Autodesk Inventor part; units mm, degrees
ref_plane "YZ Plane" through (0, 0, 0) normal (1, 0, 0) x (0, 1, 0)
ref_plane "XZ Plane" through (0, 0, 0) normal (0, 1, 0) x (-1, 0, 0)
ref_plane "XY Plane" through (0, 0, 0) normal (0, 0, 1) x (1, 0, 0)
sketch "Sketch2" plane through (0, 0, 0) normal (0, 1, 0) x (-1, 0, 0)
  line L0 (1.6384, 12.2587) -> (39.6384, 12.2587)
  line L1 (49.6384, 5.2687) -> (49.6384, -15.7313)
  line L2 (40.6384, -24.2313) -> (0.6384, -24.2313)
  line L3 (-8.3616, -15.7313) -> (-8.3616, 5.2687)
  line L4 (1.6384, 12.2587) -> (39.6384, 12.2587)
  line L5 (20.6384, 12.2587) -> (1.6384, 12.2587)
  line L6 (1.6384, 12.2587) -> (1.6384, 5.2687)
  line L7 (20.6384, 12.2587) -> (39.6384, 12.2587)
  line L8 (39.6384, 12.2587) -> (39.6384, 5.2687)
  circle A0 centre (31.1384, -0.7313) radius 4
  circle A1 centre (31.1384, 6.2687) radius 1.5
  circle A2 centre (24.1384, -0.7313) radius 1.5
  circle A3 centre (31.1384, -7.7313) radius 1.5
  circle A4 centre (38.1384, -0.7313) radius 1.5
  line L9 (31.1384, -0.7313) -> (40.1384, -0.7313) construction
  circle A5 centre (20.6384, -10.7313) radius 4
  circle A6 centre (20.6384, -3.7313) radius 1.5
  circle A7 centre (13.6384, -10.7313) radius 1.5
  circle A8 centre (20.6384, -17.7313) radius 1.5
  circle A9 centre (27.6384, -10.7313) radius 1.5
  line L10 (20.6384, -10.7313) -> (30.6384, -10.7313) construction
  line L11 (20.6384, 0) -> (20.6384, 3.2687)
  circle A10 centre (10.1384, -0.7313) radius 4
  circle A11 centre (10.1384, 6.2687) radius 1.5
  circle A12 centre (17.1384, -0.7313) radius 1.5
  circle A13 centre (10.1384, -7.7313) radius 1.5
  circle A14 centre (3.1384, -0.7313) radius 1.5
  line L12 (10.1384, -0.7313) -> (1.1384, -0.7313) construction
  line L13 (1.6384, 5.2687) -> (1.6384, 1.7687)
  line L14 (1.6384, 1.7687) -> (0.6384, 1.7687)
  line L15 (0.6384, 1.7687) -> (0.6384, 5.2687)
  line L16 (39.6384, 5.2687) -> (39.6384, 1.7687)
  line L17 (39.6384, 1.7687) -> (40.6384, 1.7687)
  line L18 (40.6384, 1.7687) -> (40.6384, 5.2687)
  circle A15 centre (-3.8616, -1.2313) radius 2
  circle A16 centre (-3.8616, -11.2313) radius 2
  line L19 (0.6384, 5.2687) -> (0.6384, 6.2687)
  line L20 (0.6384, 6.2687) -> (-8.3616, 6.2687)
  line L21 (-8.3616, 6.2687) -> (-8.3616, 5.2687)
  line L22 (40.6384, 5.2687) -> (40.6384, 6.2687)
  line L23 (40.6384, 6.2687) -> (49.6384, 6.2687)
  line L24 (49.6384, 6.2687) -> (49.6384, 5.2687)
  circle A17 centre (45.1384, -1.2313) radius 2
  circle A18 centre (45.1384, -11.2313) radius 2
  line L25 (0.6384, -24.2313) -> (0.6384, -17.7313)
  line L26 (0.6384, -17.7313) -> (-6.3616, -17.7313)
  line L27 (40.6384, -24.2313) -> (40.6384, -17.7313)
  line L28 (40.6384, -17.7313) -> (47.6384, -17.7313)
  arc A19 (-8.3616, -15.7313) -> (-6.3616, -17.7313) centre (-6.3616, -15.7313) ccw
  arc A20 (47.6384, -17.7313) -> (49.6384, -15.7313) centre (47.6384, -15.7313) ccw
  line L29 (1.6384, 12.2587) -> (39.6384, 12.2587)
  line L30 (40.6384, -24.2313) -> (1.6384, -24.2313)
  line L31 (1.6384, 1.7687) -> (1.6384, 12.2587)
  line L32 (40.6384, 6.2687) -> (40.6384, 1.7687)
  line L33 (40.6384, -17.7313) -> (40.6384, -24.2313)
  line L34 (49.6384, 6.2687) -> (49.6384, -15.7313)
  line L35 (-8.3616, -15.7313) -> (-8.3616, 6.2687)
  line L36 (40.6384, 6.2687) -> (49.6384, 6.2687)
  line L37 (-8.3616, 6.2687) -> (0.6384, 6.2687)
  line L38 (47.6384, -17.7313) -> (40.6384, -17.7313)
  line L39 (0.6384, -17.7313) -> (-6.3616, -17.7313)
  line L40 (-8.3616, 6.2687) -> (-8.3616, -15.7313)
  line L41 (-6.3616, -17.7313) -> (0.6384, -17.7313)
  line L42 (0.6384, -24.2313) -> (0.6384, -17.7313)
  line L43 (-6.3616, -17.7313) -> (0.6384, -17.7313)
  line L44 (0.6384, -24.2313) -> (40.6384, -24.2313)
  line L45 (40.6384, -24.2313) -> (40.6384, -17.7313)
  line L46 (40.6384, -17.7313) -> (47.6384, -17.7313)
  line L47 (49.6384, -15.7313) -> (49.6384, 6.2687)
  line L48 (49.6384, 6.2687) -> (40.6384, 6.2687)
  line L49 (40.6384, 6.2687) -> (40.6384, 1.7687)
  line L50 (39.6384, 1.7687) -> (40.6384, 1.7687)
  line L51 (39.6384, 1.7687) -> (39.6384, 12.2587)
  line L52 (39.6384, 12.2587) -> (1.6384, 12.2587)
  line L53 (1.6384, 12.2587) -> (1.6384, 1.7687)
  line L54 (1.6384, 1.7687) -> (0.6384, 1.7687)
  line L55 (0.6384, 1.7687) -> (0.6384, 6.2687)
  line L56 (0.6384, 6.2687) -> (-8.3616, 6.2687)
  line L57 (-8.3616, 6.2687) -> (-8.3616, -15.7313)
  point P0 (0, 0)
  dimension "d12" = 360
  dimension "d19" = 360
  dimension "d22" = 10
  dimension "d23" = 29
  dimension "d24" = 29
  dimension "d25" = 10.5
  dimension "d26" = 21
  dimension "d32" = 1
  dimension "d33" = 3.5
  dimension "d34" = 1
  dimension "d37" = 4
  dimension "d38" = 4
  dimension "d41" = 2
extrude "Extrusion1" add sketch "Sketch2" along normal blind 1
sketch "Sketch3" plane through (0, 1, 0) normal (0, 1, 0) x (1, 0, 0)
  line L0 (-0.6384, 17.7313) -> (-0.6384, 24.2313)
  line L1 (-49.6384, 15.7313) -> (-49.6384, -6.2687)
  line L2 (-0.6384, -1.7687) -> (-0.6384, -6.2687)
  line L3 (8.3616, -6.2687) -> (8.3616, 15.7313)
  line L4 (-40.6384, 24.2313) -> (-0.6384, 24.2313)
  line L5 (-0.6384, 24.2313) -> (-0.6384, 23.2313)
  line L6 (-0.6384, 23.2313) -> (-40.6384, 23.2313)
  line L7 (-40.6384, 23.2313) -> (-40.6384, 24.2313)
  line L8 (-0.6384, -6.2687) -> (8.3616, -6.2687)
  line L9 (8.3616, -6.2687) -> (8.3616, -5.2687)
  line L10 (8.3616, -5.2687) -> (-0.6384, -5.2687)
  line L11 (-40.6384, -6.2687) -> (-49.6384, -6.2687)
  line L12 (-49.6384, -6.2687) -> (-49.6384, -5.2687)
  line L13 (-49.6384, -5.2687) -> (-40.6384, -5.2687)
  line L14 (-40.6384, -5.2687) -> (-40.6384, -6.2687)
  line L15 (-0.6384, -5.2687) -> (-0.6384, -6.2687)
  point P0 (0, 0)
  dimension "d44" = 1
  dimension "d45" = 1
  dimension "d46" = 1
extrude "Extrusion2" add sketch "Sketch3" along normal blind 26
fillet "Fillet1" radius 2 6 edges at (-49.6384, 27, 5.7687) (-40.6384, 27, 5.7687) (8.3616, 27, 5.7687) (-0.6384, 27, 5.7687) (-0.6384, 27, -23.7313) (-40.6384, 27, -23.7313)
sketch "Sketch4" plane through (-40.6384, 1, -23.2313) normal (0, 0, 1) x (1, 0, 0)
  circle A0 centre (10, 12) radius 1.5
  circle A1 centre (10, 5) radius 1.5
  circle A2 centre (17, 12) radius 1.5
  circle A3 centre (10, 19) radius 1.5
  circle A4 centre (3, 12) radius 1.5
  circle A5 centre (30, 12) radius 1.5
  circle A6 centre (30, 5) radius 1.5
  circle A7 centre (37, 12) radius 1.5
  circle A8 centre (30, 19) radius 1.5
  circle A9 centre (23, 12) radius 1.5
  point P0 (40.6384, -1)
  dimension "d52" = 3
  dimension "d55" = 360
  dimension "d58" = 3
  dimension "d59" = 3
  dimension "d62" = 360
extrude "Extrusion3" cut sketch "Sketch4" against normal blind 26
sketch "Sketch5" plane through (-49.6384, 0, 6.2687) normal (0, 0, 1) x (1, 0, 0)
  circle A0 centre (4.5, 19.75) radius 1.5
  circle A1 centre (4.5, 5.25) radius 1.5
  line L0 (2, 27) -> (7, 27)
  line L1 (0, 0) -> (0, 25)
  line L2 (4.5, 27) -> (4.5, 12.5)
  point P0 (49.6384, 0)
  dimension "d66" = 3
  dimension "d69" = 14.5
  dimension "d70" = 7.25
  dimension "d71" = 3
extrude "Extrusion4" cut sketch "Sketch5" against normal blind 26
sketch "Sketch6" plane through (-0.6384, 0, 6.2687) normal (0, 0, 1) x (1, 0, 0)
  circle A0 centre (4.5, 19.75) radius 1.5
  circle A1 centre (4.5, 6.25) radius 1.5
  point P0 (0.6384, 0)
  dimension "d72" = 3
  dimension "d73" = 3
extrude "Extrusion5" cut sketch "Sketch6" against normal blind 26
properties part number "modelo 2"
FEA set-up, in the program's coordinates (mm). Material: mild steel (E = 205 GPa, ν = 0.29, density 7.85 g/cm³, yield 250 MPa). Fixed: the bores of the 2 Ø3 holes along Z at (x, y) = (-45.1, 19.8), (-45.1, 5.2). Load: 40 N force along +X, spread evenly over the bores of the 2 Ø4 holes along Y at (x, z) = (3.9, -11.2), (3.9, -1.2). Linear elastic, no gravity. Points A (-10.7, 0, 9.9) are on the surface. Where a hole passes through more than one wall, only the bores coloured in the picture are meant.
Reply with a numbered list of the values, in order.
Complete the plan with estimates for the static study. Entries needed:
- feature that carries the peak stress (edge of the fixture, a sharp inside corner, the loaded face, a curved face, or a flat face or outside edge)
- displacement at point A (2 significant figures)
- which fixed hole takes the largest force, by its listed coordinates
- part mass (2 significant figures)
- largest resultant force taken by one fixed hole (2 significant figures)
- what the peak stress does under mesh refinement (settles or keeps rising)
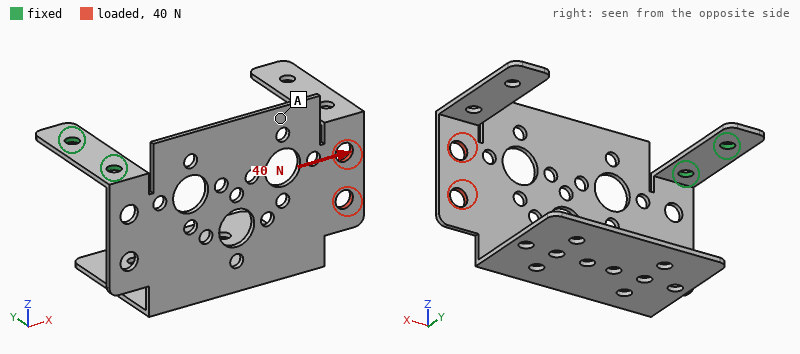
1. edge of the fixture
2. 0.19 mm
3. (-45.1, 5.2)
4. 23 g
5. 45 N
6. keeps rising
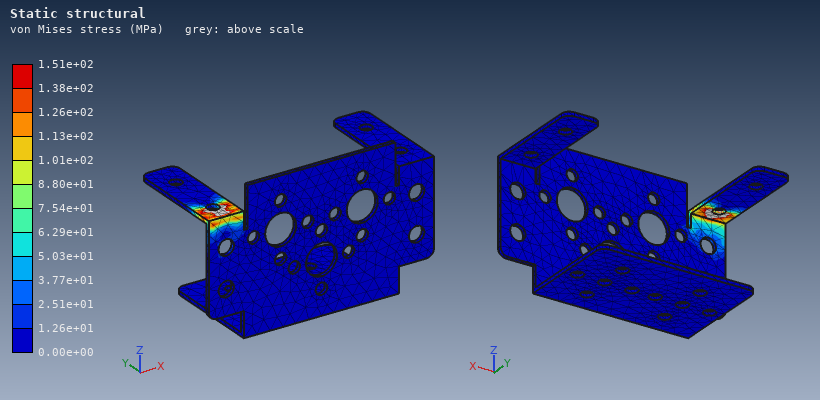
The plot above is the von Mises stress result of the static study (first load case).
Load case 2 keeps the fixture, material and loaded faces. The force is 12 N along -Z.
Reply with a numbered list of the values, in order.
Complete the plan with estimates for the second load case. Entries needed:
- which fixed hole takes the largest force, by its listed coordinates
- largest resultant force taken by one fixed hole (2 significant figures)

1. (-45.1, 5.2)
2. 12 N
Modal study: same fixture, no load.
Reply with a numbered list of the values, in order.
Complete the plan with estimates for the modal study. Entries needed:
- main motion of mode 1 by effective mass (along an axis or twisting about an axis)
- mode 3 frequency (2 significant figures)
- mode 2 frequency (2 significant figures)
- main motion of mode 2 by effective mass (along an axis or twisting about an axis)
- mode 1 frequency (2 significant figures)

1. along Y
2. 310 Hz
3. 190 Hz
4. along Z
5. 110 Hz
